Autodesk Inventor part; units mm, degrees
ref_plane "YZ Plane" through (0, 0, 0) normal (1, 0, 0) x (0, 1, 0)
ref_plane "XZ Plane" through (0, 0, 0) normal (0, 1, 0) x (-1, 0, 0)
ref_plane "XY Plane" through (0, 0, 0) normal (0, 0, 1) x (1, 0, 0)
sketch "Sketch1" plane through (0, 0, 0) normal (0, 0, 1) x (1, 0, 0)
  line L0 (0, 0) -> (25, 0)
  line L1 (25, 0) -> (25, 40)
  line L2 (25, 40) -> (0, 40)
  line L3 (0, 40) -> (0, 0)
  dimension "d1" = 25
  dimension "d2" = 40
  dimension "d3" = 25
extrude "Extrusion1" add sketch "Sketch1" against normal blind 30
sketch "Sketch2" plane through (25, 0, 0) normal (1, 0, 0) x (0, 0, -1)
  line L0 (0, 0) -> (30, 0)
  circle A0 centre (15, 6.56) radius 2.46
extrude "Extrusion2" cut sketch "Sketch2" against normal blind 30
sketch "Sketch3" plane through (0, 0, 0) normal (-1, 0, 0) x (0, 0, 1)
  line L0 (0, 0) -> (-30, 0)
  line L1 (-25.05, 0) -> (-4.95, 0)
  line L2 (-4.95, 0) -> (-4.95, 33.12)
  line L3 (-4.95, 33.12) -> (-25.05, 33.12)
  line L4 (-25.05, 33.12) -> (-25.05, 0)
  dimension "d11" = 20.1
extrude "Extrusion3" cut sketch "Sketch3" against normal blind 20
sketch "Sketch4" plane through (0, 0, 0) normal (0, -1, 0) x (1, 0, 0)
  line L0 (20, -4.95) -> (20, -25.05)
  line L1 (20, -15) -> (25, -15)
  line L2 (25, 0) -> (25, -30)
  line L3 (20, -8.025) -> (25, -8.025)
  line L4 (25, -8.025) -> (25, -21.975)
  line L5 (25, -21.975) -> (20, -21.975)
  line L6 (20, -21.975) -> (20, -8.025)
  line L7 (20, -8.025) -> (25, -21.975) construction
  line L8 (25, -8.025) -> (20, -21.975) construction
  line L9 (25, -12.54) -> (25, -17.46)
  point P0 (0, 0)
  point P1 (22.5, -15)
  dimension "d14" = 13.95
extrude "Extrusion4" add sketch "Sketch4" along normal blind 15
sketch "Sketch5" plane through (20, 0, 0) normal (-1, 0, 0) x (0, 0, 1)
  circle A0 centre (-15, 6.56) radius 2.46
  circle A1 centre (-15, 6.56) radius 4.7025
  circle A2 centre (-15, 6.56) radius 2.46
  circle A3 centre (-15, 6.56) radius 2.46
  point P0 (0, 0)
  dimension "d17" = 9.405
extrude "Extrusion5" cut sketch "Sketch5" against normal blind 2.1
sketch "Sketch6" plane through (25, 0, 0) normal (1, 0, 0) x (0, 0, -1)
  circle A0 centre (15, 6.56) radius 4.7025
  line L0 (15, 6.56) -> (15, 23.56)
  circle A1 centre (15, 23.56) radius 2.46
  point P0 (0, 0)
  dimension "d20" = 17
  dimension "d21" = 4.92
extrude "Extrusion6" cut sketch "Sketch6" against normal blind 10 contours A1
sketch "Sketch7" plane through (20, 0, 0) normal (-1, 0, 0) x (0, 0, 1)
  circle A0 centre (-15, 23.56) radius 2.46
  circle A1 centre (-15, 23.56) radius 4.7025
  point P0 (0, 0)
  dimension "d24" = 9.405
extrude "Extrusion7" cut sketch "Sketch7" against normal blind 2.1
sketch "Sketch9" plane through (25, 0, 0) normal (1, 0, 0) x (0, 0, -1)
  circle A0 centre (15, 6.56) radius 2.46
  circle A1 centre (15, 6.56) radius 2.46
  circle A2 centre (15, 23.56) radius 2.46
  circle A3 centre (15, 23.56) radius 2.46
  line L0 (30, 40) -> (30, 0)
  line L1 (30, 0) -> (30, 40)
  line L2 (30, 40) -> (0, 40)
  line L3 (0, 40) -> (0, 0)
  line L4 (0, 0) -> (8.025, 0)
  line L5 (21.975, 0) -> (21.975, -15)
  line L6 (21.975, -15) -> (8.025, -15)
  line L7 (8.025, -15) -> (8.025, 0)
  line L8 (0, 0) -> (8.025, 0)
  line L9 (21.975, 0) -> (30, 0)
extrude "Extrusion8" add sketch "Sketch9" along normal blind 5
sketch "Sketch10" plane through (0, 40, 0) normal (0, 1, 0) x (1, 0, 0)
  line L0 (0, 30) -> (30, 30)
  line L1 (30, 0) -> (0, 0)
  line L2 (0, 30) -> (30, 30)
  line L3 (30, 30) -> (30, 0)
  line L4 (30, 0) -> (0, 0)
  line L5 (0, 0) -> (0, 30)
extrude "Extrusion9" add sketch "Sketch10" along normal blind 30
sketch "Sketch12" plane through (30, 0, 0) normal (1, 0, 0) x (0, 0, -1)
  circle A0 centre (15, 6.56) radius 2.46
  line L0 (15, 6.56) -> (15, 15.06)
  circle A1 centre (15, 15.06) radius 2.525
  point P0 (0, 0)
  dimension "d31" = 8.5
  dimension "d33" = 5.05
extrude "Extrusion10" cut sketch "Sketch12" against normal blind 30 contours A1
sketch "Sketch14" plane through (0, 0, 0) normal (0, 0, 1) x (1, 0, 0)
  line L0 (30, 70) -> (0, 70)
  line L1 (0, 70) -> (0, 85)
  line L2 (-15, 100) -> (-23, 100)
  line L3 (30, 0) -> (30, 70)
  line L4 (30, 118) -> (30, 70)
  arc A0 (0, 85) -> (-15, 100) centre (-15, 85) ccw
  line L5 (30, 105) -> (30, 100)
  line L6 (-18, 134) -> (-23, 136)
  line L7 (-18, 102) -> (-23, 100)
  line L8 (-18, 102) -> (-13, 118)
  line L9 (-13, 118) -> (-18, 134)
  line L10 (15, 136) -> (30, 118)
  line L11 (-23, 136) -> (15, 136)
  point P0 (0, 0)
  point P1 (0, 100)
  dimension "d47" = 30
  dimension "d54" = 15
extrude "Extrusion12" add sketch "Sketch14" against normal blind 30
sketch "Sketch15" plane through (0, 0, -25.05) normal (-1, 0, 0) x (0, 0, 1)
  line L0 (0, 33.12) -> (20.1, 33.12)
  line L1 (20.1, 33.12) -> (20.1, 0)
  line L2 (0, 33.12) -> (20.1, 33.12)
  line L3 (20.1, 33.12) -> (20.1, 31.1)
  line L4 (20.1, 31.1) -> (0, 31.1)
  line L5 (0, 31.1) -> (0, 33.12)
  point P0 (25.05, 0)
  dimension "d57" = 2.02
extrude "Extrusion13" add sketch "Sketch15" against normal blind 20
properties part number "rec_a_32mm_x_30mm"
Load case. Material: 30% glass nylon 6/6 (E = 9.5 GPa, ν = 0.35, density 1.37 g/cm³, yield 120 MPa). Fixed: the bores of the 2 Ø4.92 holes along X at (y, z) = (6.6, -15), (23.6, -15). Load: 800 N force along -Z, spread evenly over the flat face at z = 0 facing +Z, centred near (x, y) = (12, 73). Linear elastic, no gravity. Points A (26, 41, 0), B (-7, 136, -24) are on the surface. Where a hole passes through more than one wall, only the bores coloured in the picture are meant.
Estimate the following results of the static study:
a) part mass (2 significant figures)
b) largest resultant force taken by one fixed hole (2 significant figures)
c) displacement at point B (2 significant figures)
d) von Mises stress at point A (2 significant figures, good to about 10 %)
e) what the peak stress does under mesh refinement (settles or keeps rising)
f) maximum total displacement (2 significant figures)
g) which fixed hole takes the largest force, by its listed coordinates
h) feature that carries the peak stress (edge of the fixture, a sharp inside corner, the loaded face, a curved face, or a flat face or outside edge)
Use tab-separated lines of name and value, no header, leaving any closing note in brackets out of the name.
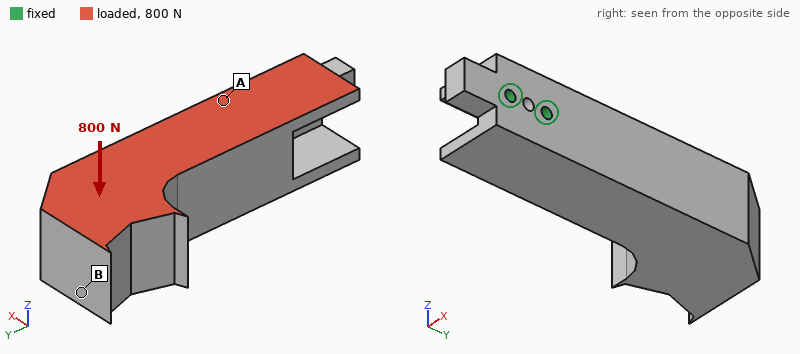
part mass	170 g
largest resultant force taken by one fixed hole	2.5 kN
displacement at point B	0.74 mm
von Mises stress at point A	8.3 MPa
what the peak stress does under mesh refinement	keeps rising
maximum total displacement	0.79 mm
which fixed hole takes the largest force, by its listed coordinates	(23.6, -15)
feature that carries the peak stress	edge of the fixture
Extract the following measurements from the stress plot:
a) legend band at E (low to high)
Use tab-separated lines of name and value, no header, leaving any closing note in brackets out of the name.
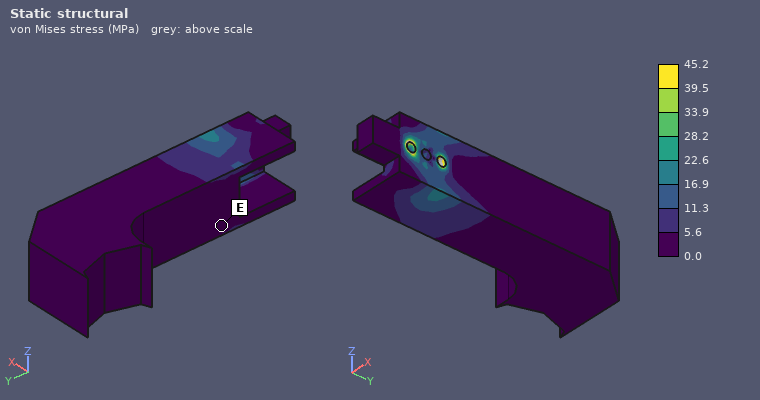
legend band at E	0.0 to 5.6 MPa
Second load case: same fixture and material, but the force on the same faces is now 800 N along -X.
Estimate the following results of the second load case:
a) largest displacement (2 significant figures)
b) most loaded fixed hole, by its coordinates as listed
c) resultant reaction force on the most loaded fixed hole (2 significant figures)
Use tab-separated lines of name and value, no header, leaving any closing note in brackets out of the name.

largest displacement	1.1 mm
most loaded fixed hole, by its coordinates as listed	(23.6, -15)
resultant reaction force on the most loaded fixed hole	2.3 kN
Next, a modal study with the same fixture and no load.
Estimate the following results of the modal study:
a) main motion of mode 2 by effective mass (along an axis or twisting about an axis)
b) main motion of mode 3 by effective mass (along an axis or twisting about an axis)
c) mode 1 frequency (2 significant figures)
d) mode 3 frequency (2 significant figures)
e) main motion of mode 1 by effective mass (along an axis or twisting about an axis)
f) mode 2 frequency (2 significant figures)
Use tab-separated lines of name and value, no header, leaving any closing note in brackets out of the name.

main motion of mode 2 by effective mass	along Z
main motion of mode 3 by effective mass	twisting about Y
mode 1 frequency	400 Hz
mode 3 frequency	1400 Hz
main motion of mode 1 by effective mass	along X
mode 2 frequency	470 Hz
